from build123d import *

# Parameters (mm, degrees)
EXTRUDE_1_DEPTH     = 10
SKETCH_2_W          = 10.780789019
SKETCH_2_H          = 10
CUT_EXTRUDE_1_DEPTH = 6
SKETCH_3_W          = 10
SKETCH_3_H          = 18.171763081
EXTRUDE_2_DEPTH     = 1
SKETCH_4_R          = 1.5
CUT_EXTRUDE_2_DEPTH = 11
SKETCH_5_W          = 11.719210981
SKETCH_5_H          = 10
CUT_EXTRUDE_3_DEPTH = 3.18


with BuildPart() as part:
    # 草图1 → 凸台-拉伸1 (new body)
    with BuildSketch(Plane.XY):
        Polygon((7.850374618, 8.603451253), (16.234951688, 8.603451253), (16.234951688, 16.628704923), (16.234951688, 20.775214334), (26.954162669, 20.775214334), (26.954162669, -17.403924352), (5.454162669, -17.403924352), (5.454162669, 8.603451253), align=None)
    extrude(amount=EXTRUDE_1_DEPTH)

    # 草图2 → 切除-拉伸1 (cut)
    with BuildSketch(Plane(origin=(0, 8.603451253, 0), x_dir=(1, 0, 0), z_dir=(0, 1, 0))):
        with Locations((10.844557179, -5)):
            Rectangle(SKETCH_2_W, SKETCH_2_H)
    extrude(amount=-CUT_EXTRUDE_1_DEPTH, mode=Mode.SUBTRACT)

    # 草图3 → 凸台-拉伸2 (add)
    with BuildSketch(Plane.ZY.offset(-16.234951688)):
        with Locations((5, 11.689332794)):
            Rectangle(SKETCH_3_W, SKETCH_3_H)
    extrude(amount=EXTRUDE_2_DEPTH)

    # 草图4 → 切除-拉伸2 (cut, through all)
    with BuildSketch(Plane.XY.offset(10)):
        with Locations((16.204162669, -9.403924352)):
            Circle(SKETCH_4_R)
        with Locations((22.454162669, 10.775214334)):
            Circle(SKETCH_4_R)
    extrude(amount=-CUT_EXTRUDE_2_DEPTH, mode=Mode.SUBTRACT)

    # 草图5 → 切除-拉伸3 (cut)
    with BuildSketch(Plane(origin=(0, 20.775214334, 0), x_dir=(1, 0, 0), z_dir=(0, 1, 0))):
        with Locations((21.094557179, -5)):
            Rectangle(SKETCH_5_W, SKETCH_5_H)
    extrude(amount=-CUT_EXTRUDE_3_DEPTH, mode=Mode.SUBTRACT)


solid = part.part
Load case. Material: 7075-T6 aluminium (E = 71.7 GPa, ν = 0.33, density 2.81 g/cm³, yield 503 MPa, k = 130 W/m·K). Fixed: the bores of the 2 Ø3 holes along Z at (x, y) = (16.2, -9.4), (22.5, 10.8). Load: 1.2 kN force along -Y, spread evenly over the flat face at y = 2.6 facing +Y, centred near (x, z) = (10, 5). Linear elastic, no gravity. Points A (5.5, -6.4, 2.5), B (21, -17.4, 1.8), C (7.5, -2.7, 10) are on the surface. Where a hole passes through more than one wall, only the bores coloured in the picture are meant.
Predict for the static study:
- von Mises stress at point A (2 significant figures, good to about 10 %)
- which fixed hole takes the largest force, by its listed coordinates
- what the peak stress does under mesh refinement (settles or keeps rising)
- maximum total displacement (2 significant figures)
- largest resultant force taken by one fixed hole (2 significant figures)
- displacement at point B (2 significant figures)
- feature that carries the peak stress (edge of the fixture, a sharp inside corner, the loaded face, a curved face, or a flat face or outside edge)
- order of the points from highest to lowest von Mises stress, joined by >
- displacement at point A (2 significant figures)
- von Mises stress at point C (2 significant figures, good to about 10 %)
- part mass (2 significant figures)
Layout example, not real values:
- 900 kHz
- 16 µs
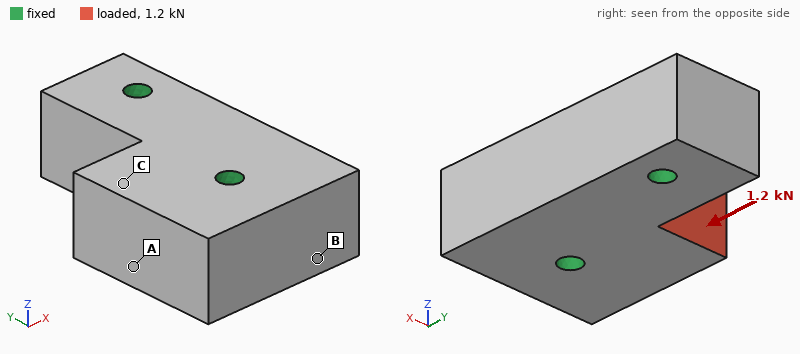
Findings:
- 6.4 MPa
- (16.2, -9.4)
- keeps rising
- 5.3 µm
- 1.1 kN
- 1.1 µm
- edge of the fixture
- C > A > B
- 3.3 µm
- 10 MPa
- 17 g
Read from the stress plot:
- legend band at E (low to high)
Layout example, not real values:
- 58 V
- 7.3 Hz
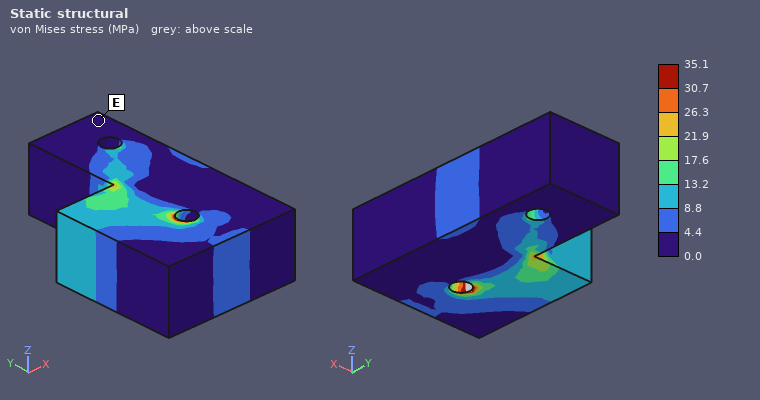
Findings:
- 0.0 to 4.4 MPa
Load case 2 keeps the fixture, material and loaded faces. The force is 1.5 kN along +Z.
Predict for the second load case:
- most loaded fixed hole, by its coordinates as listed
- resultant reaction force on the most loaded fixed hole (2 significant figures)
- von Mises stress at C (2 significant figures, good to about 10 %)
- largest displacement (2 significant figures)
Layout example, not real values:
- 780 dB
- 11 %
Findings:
- (16.2, -9.4)
- 970 N
- 29 MPa
- 24 µm
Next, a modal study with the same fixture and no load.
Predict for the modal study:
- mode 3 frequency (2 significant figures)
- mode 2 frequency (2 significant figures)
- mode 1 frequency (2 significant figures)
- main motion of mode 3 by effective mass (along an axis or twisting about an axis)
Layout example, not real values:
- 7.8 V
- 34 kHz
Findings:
- 43 kHz
- 35 kHz
- 33 kHz
- along Z
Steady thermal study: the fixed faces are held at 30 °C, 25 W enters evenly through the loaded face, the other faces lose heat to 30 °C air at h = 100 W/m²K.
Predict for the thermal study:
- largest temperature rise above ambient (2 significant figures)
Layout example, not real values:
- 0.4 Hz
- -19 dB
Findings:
- 19 K
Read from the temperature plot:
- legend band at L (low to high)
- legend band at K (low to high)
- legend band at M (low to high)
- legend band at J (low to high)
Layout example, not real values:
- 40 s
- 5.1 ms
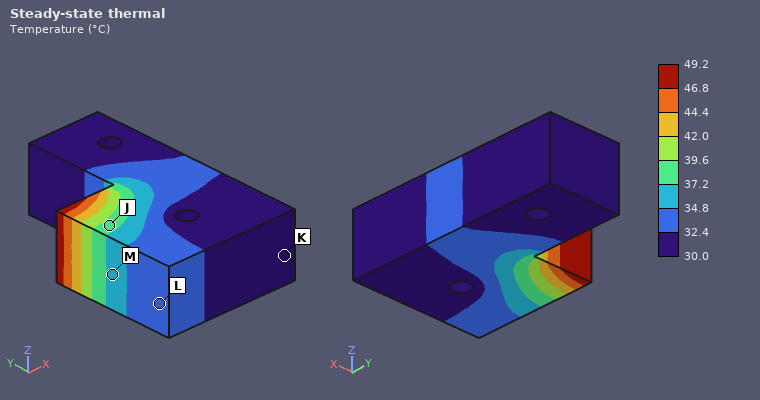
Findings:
- 32.4 to 34.8 °C
- 30.0 to 32.4 °C
- 34.8 to 37.2 °C
- 37.2 to 39.6 °C
